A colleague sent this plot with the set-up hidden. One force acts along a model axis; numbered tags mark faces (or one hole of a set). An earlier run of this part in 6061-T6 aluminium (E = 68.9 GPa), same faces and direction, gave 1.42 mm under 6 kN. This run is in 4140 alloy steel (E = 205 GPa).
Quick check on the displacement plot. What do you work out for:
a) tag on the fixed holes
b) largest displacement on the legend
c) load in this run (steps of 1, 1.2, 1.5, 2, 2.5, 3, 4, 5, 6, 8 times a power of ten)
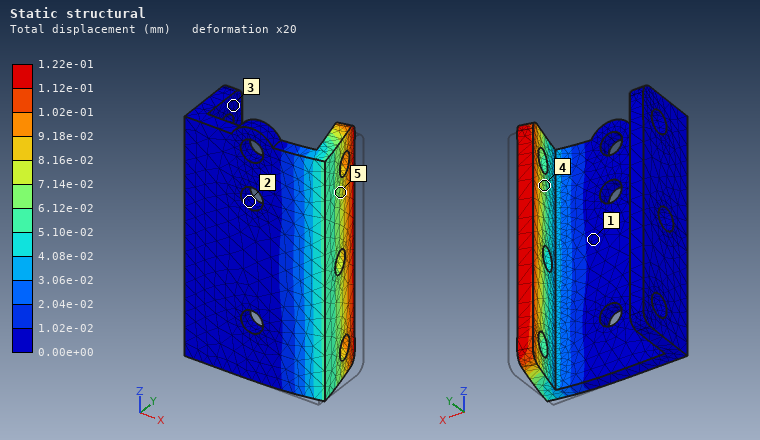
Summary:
2
1.22e-01 mm
1.5 kN
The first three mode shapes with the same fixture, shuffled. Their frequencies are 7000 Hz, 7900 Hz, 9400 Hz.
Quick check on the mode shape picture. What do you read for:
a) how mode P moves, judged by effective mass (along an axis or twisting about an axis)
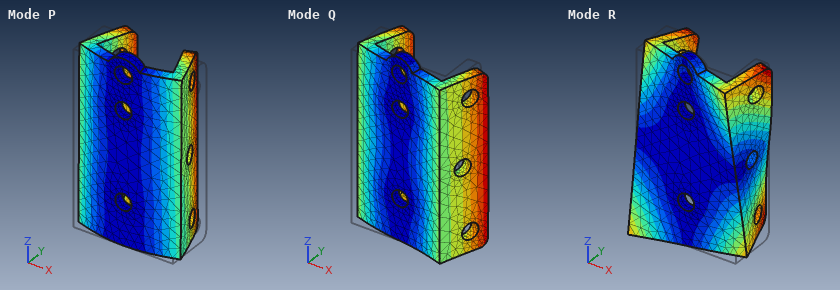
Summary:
along Y
